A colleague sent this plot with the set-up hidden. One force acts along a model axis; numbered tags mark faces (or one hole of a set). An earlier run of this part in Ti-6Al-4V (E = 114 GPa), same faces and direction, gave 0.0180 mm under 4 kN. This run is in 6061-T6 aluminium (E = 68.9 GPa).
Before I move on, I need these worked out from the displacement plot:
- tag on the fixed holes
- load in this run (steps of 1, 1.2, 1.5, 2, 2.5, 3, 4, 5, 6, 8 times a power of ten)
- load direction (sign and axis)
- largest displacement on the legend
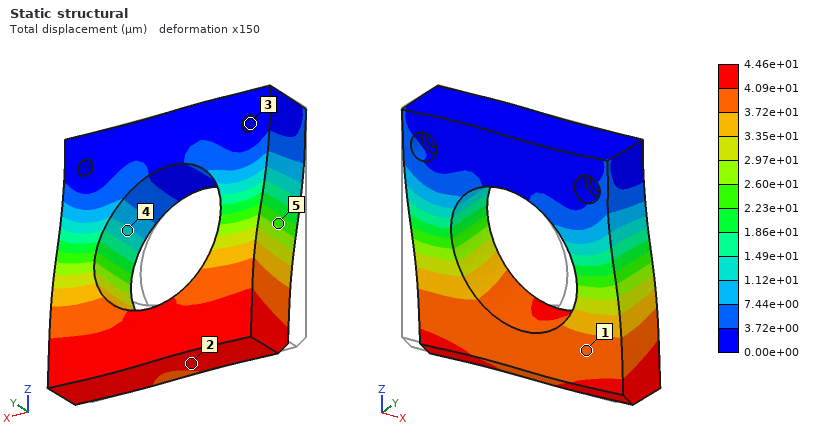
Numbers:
3
6 kN
+X
4.46e+01 µm
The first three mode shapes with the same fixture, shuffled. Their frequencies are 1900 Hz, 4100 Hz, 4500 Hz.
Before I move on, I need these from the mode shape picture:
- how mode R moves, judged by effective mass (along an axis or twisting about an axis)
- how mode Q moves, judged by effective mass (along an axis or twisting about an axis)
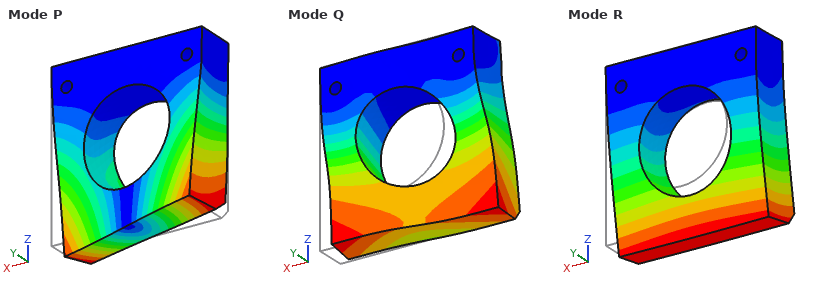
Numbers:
along Y
along X
